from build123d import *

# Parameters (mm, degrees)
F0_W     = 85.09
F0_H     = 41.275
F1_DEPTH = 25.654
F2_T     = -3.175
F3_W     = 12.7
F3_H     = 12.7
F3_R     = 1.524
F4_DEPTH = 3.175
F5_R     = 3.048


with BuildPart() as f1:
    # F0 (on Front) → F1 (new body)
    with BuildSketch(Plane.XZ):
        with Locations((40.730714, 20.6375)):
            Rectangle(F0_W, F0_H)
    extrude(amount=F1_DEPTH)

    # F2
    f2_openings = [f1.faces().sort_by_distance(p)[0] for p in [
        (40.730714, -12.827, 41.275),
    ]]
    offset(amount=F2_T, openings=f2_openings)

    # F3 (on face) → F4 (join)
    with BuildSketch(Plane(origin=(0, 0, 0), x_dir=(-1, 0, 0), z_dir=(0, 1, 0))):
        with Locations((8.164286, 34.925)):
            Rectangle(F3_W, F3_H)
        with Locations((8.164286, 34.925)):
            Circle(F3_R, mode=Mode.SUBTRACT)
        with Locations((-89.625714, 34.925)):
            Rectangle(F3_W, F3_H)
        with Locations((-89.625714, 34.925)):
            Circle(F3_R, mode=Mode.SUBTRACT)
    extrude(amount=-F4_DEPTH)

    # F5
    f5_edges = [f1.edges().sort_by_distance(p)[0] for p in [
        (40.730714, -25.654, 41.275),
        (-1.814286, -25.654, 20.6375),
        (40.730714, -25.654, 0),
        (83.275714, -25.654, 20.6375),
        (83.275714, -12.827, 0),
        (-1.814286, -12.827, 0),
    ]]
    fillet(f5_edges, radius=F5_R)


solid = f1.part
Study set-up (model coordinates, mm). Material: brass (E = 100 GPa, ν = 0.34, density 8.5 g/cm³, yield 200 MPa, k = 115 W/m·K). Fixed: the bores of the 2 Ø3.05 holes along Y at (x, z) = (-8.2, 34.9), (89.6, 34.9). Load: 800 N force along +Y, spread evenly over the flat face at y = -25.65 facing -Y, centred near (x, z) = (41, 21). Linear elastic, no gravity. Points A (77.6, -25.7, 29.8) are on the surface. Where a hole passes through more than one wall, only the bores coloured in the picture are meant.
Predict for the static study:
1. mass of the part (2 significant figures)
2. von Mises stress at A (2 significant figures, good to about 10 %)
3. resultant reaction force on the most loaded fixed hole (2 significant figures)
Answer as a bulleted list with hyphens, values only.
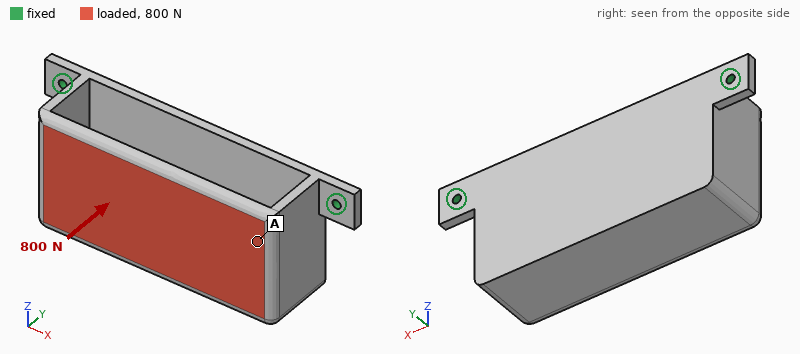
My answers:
- 280 g
- 28 MPa
- 410 N
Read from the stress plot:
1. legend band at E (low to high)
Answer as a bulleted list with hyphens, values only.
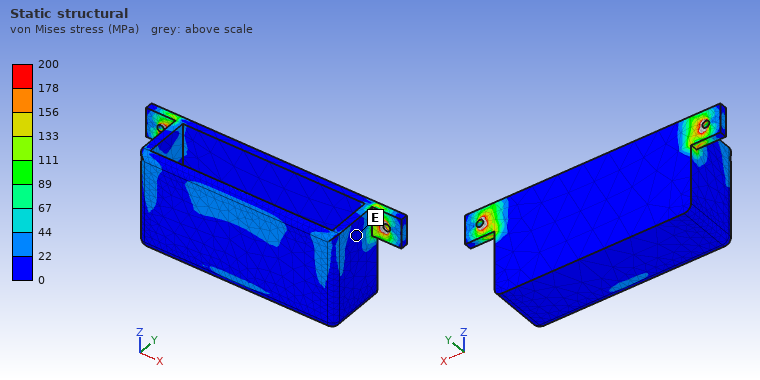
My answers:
- 0 to 22 MPa
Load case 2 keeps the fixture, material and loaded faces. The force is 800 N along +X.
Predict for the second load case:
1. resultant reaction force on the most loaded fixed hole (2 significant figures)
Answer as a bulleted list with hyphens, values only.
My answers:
- 460 N
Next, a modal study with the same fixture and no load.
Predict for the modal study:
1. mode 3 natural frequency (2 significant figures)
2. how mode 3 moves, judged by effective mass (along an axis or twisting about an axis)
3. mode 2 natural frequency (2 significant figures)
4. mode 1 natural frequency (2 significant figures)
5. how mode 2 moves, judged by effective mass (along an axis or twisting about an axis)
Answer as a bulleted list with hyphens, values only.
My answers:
- 1900 Hz
- along Y
- 1300 Hz
- 470 Hz
- along X
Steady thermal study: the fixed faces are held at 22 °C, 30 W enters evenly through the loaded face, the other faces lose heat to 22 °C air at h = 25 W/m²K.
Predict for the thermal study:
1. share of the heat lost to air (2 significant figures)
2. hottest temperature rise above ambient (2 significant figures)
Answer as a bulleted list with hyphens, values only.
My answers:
- 42 %
- 43 K
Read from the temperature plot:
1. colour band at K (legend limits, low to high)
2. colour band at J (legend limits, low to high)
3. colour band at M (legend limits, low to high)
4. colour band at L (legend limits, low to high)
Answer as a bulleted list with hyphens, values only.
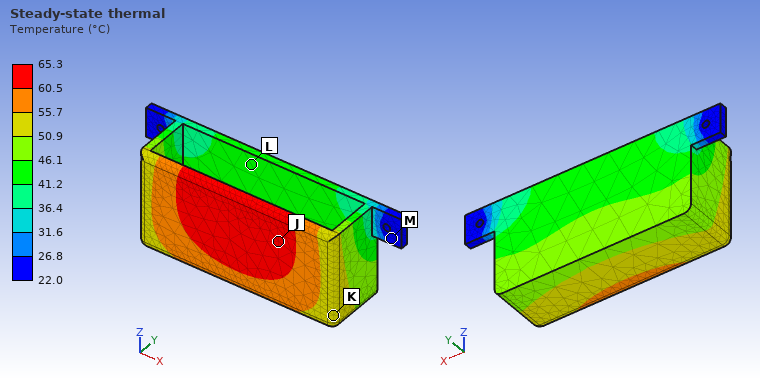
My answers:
- 50.9 to 55.7 °C
- 60.5 to 65.3 °C
- 22.0 to 26.8 °C
- 41.2 to 46.1 °C
